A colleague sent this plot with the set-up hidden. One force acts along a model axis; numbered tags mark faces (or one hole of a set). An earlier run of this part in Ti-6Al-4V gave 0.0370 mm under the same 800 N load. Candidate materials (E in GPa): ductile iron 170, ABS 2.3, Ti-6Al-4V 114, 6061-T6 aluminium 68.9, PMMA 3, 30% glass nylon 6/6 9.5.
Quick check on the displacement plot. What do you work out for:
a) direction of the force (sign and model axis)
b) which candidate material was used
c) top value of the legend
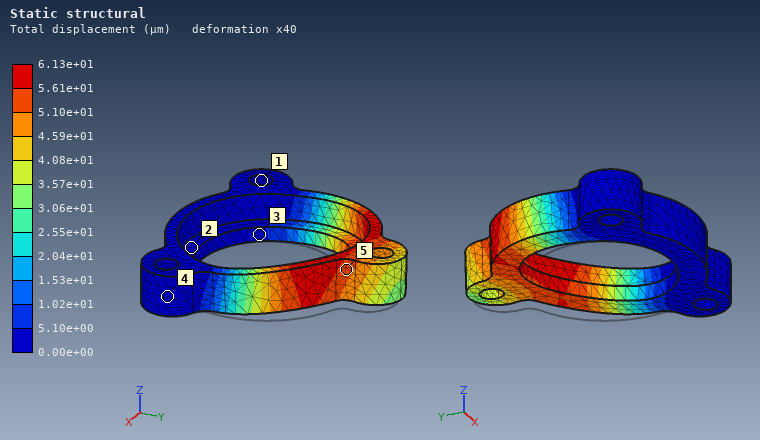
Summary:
-X
6061-T6 aluminium
6.13e+01 µm
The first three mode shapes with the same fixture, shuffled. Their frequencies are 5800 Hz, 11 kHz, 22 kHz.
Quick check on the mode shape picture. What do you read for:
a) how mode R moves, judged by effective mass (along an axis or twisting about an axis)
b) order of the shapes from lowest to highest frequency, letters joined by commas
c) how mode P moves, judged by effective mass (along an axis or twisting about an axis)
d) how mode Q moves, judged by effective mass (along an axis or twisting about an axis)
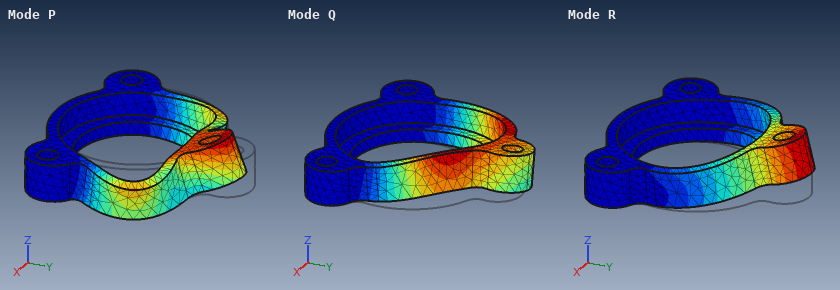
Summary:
along Z
R, Q, P
along Y
along X
